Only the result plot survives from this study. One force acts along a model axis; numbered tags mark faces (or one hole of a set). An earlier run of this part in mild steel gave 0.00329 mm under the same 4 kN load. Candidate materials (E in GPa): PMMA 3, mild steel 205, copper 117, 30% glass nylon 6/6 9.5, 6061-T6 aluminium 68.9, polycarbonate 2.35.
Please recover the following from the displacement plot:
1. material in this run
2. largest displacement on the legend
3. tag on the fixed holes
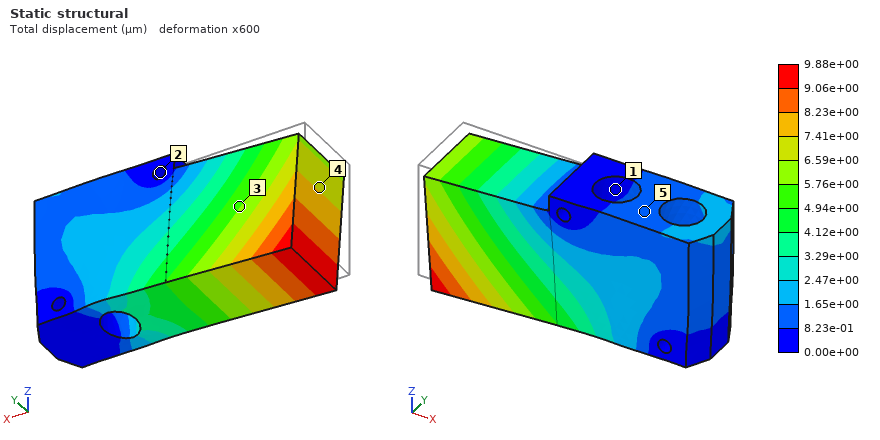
6061-T6 aluminium
9.88e+00 µm
2
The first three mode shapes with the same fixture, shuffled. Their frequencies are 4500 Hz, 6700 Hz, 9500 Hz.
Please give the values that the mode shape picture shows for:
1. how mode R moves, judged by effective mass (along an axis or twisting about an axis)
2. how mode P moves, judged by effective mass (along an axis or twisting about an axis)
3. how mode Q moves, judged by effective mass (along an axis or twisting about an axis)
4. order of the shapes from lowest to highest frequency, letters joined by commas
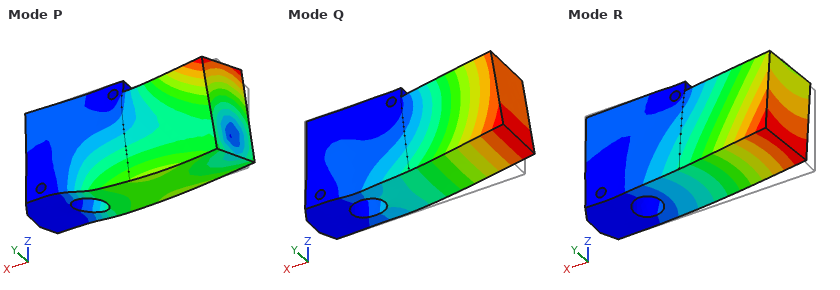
along Y
twisting about X
along Z
R, Q, P
